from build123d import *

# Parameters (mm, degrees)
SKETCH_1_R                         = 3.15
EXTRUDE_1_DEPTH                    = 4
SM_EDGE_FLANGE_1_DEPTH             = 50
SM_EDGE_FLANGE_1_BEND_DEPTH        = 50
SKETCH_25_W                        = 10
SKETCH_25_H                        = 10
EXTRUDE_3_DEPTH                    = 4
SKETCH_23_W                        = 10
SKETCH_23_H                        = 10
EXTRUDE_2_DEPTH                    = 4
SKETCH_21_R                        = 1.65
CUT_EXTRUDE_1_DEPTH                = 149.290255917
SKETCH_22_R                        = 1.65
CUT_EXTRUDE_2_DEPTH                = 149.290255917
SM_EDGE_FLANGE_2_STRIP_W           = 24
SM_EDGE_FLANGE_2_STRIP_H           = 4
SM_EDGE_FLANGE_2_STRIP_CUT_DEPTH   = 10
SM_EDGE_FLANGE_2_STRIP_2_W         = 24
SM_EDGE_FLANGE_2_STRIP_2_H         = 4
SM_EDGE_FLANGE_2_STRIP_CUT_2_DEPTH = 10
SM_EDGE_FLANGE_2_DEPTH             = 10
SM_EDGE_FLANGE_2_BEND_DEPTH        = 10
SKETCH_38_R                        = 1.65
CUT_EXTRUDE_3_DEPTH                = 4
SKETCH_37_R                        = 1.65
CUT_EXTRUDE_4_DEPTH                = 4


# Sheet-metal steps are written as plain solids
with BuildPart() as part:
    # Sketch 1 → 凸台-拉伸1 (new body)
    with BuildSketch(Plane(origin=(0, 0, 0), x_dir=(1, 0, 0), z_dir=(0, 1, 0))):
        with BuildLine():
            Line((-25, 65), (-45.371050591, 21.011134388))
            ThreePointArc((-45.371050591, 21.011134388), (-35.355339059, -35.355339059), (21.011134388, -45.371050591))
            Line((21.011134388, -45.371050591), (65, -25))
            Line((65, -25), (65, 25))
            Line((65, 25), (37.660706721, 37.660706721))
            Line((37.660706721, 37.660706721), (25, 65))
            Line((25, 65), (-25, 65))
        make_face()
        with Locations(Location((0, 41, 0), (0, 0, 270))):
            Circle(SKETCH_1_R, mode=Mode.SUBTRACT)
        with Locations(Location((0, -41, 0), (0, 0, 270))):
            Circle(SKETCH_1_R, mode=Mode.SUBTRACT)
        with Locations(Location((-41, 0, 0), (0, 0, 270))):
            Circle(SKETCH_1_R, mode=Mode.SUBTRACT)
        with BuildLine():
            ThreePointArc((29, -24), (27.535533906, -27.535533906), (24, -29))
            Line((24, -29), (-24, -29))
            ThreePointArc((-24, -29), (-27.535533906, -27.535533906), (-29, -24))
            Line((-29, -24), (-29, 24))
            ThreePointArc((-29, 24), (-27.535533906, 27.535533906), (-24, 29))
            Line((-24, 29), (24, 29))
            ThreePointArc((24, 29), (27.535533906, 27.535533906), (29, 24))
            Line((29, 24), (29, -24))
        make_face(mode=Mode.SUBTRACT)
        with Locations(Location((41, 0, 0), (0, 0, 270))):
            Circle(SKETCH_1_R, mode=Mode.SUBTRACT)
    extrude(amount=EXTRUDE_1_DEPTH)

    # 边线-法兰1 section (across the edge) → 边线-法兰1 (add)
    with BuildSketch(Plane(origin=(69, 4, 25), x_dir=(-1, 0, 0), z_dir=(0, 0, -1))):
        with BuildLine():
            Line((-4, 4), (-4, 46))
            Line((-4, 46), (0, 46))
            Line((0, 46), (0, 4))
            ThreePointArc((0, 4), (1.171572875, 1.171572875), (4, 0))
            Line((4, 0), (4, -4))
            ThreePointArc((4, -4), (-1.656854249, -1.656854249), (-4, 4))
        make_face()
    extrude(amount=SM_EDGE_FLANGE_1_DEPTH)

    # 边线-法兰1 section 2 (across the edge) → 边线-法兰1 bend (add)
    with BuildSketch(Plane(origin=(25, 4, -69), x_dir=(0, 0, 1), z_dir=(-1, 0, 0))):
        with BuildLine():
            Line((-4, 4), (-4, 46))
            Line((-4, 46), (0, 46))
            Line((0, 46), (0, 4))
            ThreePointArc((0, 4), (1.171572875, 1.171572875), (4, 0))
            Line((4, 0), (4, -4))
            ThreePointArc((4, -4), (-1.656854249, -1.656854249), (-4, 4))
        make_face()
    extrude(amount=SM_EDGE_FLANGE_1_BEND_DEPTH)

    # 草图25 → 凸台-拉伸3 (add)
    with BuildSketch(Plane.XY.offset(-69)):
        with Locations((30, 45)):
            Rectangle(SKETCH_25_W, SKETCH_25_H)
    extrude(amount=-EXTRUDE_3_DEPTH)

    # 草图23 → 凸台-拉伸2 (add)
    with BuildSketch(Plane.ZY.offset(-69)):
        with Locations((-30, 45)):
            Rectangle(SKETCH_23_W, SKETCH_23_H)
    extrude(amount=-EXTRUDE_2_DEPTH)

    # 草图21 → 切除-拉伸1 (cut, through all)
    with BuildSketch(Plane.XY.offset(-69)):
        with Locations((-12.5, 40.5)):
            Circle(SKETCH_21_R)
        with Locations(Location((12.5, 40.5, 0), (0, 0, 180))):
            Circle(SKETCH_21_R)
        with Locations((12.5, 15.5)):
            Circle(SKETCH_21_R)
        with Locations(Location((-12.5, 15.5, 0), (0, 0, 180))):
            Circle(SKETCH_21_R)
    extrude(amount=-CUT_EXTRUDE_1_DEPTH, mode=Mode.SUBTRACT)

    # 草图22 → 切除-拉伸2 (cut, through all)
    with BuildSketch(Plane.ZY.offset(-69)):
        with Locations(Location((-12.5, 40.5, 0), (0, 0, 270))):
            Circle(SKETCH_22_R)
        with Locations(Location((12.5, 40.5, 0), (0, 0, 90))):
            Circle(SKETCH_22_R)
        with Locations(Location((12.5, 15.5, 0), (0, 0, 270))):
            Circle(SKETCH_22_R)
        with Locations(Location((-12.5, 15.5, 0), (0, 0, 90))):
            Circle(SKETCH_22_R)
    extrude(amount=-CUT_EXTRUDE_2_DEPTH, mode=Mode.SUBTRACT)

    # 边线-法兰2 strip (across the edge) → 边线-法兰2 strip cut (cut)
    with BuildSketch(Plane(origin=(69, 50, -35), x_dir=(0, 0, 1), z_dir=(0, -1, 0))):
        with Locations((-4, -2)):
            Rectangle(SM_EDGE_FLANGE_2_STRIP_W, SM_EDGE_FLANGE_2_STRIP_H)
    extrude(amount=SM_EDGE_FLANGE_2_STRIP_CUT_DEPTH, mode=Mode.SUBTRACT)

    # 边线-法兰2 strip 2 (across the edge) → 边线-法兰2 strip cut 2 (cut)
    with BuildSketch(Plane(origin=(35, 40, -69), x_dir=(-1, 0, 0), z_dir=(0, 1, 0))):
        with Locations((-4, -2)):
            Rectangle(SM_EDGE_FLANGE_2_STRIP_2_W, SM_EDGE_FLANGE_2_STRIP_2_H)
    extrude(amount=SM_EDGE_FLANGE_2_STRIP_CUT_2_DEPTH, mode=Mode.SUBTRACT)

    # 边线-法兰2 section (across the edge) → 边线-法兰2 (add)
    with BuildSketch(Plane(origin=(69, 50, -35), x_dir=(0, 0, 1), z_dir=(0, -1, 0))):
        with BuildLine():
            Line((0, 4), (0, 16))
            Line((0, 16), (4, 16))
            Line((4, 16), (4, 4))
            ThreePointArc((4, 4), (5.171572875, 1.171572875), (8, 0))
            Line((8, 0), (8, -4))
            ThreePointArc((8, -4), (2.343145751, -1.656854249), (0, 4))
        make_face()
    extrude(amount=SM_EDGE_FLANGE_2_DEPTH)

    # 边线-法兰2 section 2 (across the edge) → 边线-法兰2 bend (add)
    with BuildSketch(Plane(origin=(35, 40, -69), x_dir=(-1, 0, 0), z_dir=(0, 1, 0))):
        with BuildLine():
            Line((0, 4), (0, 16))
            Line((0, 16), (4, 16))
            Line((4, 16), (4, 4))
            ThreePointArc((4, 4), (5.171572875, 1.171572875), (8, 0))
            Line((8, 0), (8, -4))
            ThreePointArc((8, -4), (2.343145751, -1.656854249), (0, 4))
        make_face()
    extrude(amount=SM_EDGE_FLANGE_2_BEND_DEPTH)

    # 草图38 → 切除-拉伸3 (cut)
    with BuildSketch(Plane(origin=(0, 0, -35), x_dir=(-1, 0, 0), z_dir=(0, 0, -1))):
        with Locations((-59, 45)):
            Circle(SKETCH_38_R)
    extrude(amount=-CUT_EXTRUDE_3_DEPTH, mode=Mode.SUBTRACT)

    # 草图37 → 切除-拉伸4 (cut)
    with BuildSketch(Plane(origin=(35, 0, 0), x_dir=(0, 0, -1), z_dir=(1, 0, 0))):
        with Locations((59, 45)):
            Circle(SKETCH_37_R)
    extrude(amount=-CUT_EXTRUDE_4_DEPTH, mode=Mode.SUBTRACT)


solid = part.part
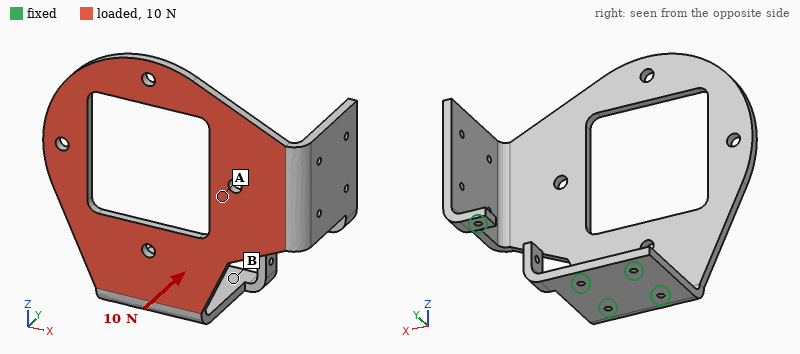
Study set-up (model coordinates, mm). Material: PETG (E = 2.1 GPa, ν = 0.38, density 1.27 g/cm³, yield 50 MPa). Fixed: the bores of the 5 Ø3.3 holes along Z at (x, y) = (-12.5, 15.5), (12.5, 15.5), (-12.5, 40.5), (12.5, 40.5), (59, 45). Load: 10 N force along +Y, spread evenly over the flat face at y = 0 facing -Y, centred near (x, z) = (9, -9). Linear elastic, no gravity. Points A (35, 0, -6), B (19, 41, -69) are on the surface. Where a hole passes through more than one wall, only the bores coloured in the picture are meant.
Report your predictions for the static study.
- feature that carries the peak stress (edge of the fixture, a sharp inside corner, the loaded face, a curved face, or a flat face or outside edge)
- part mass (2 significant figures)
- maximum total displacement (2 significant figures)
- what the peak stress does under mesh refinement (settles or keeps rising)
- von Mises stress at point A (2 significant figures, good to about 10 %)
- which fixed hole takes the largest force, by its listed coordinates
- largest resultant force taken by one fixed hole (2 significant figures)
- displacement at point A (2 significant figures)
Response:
edge of the fixture
62 g
1.8 mm
keeps rising
0.74 MPa
(12.5, 15.5)
19 N
0.44 mm
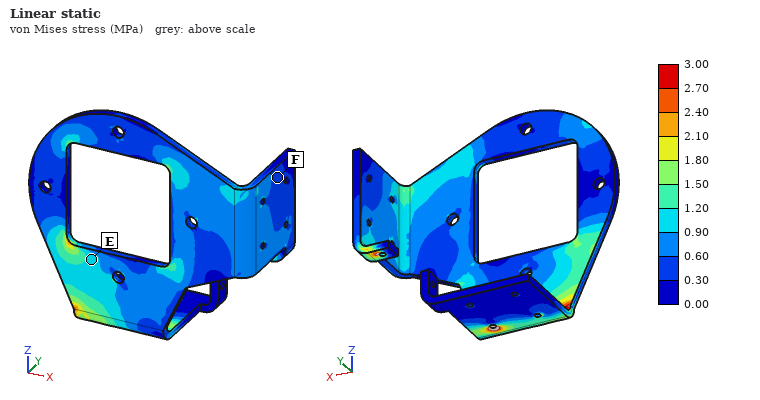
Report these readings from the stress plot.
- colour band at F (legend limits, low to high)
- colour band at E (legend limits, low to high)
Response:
0.30 to 0.60 MPa
0.90 to 1.20 MPa
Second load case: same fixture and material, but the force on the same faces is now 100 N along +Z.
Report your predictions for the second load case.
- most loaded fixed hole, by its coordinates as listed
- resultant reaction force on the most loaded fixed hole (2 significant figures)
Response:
(12.5, 15.5)
95 N
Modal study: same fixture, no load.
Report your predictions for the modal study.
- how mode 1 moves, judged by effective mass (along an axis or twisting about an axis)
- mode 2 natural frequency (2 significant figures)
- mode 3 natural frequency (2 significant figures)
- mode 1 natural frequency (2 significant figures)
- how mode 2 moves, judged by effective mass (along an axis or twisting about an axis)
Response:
along Y
140 Hz
250 Hz
81 Hz
along X
